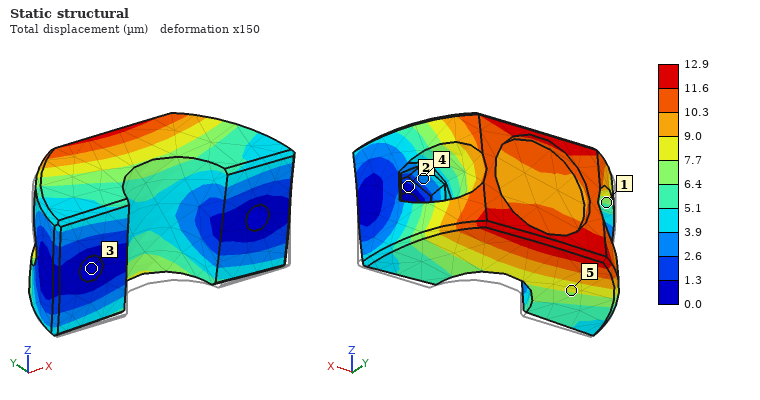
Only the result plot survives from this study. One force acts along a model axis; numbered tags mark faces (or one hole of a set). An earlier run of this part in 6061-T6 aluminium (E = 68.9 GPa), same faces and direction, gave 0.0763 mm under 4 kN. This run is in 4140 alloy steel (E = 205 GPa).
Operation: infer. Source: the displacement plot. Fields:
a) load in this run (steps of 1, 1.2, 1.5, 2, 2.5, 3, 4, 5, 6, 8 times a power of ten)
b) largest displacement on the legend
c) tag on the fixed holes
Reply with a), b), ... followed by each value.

a) 2 kN
b) 12.9 µm
c) 3
